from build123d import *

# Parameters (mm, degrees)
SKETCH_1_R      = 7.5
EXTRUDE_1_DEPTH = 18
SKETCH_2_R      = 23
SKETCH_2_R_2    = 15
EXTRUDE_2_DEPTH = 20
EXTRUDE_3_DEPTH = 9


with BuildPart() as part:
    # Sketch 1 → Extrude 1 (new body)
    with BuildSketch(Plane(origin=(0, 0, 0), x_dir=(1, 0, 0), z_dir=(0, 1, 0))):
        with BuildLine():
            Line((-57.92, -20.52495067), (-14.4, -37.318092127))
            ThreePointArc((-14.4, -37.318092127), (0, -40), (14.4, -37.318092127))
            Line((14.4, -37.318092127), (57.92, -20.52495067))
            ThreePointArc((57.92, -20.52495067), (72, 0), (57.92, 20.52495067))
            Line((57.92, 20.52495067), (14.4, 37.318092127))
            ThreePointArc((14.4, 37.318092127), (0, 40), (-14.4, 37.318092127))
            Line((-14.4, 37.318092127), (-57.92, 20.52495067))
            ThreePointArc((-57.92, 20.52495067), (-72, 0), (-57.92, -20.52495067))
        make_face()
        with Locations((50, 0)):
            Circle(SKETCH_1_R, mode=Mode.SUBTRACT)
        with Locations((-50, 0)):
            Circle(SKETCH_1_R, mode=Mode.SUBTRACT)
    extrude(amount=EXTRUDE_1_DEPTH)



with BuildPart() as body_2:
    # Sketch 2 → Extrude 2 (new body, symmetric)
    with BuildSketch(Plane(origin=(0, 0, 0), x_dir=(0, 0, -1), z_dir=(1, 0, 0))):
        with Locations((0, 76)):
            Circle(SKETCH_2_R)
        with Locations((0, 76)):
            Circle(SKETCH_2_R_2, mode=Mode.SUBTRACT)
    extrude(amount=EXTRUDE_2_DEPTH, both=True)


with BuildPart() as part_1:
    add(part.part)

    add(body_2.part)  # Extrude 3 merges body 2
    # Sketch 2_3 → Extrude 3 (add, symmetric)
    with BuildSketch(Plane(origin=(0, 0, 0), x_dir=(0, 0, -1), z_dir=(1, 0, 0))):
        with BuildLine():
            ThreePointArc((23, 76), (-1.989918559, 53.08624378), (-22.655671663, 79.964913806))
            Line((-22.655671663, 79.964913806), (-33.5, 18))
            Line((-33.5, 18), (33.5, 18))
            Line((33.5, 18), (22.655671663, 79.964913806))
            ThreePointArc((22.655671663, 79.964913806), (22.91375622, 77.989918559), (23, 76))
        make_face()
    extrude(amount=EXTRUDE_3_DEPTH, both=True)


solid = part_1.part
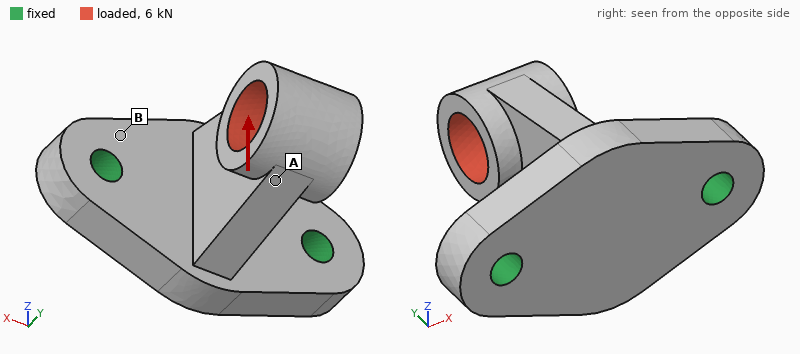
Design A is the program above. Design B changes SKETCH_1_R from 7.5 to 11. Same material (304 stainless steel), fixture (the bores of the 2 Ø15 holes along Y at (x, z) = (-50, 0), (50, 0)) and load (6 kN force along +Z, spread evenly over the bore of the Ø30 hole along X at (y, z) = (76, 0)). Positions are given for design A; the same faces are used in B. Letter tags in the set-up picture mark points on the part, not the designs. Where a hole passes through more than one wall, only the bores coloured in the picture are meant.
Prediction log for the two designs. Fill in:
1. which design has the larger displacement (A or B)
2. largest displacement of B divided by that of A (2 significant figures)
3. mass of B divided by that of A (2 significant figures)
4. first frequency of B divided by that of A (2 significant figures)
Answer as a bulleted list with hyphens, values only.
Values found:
- A
- 0.83
- 0.97
- 1.0
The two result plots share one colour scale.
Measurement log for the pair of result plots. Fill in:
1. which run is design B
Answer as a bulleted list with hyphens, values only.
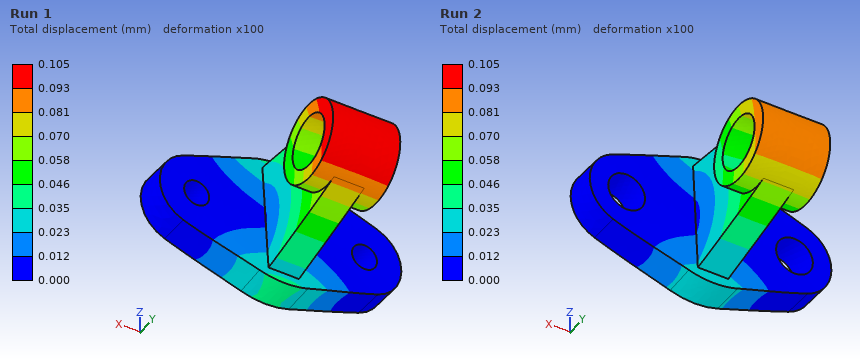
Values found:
- Run 2
